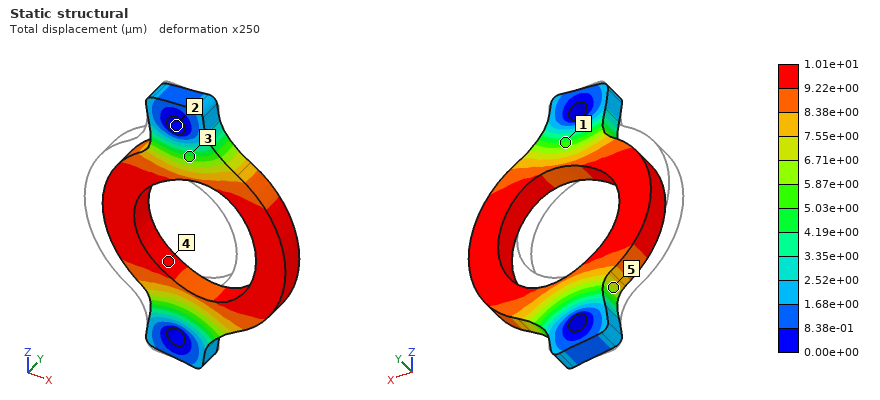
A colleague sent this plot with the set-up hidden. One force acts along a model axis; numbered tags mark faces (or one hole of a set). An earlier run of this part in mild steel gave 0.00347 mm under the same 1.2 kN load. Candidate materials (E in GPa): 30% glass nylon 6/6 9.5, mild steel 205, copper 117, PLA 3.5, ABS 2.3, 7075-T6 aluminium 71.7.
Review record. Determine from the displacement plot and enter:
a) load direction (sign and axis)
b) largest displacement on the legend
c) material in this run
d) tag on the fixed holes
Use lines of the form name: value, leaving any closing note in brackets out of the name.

load direction: +X
largest displacement on the legend: 1.01e+01 µm
material in this run: 7075-T6 aluminium
tag on the fixed holes: 2
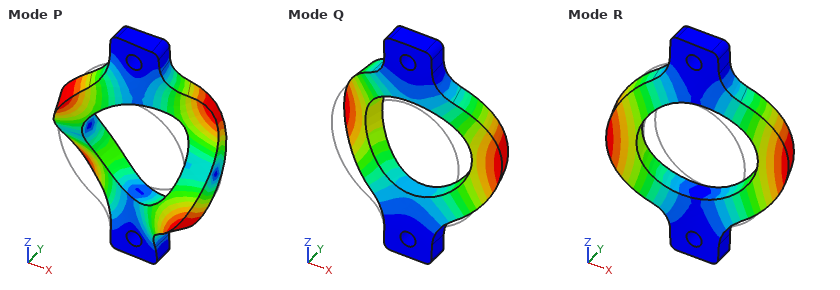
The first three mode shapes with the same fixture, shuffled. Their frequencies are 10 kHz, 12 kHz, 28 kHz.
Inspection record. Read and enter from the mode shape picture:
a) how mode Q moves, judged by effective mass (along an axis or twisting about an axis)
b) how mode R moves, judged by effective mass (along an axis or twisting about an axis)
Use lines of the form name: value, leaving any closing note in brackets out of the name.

how mode Q moves, judged by effective mass: along Y
how mode R moves, judged by effective mass: twisting about Z
